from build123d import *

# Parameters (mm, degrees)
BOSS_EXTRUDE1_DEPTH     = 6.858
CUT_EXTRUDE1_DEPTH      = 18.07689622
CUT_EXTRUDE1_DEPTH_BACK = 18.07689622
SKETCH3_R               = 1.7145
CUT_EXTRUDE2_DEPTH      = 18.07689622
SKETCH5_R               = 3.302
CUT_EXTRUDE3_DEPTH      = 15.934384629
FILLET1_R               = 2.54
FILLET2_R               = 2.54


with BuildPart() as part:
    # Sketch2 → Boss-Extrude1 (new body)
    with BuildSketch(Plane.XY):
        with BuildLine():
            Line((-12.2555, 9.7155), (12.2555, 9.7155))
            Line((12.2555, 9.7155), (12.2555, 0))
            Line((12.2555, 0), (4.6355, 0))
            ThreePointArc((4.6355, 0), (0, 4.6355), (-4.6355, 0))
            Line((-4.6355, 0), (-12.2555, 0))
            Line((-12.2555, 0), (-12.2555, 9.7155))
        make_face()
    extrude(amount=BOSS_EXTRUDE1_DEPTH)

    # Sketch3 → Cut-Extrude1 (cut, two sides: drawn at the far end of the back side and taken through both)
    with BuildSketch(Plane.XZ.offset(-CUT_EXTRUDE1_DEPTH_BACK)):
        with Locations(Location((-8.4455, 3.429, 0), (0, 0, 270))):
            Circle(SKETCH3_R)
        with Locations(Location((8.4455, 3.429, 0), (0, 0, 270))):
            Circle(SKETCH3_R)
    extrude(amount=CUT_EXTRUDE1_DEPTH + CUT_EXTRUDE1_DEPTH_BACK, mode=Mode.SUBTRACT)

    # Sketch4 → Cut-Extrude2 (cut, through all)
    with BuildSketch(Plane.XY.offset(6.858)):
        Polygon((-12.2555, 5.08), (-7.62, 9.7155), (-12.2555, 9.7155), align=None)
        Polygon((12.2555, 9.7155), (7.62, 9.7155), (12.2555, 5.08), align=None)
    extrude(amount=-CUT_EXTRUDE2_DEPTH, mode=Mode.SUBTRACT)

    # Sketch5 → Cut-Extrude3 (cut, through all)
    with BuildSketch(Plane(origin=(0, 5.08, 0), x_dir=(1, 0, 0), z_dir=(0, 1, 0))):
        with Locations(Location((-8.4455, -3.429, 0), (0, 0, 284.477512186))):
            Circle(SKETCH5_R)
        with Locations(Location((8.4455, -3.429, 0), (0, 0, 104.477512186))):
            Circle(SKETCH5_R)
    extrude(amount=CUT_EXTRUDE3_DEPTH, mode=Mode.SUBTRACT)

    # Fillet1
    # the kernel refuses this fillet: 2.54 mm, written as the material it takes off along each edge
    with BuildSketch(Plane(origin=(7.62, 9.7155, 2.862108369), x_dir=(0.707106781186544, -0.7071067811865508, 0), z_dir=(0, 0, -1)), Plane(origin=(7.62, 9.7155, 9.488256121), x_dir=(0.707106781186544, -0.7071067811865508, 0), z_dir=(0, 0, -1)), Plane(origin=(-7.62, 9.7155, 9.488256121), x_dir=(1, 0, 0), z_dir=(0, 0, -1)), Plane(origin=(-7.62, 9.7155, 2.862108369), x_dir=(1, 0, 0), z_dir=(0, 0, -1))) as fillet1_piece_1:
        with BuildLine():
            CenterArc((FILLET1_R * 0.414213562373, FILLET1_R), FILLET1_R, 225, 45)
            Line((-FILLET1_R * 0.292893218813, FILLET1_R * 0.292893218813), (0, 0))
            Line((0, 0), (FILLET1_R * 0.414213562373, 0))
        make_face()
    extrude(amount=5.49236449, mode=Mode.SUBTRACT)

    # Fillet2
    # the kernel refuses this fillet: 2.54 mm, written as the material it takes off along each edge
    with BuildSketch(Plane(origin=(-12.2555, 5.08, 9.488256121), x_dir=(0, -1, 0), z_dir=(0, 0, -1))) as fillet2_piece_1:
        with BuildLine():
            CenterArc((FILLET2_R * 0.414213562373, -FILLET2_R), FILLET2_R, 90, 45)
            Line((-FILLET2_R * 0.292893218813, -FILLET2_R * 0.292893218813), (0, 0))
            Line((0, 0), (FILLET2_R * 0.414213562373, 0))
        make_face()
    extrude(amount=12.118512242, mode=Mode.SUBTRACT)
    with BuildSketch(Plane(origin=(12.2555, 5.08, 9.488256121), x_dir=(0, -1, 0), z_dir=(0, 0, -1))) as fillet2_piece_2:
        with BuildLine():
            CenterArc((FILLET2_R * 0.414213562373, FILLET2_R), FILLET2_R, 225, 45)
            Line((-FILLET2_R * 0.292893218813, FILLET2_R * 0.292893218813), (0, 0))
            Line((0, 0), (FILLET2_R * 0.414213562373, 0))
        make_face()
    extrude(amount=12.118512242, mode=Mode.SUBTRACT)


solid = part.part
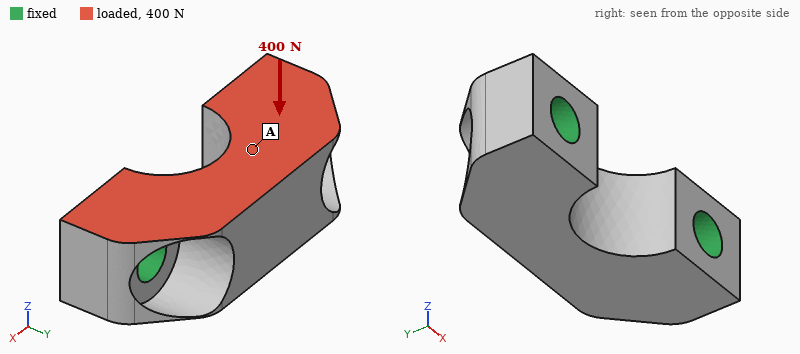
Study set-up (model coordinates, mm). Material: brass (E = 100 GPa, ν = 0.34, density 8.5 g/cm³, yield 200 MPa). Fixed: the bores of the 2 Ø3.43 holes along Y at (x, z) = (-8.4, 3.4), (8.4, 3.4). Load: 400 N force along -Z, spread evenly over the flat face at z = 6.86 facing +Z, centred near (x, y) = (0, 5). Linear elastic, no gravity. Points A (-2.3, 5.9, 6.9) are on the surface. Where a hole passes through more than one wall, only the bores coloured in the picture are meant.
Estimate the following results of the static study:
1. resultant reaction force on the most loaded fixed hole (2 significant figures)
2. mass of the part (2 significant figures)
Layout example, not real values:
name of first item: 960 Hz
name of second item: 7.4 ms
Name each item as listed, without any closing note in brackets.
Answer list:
resultant reaction force on the most loaded fixed hole: 200 N
mass of the part: 7.8 g
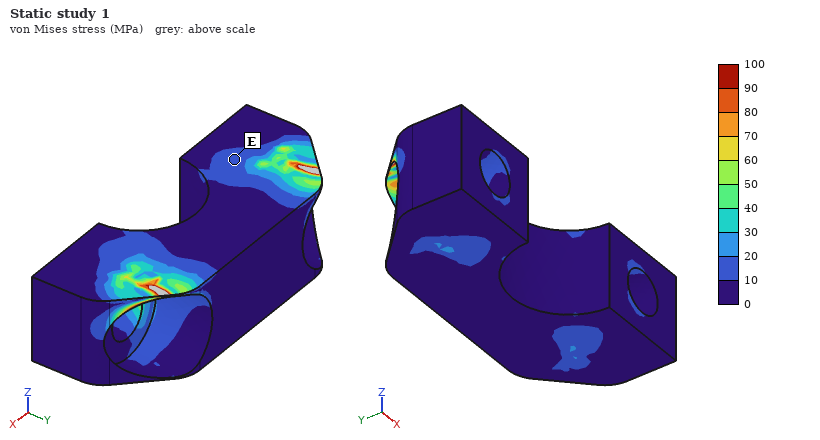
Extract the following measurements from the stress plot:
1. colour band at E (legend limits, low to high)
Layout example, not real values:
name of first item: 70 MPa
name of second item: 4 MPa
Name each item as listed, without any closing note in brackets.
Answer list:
colour band at E: 10 to 20 MPa
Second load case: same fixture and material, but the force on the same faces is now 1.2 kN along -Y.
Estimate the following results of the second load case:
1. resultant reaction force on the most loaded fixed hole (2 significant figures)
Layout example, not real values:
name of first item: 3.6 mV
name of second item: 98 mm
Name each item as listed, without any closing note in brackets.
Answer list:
resultant reaction force on the most loaded fixed hole: 610 N
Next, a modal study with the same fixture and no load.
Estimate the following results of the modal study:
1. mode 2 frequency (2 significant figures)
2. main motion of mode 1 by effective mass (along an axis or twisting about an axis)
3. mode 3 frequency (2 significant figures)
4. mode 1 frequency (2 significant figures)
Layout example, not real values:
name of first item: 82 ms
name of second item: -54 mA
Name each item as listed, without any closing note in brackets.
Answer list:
mode 2 frequency: 54 kHz
main motion of mode 1 by effective mass: along Z
mode 3 frequency: 54 kHz
mode 1 frequency: 27 kHz
